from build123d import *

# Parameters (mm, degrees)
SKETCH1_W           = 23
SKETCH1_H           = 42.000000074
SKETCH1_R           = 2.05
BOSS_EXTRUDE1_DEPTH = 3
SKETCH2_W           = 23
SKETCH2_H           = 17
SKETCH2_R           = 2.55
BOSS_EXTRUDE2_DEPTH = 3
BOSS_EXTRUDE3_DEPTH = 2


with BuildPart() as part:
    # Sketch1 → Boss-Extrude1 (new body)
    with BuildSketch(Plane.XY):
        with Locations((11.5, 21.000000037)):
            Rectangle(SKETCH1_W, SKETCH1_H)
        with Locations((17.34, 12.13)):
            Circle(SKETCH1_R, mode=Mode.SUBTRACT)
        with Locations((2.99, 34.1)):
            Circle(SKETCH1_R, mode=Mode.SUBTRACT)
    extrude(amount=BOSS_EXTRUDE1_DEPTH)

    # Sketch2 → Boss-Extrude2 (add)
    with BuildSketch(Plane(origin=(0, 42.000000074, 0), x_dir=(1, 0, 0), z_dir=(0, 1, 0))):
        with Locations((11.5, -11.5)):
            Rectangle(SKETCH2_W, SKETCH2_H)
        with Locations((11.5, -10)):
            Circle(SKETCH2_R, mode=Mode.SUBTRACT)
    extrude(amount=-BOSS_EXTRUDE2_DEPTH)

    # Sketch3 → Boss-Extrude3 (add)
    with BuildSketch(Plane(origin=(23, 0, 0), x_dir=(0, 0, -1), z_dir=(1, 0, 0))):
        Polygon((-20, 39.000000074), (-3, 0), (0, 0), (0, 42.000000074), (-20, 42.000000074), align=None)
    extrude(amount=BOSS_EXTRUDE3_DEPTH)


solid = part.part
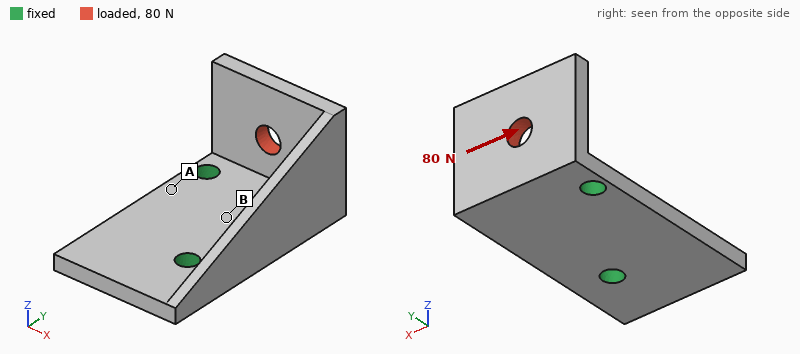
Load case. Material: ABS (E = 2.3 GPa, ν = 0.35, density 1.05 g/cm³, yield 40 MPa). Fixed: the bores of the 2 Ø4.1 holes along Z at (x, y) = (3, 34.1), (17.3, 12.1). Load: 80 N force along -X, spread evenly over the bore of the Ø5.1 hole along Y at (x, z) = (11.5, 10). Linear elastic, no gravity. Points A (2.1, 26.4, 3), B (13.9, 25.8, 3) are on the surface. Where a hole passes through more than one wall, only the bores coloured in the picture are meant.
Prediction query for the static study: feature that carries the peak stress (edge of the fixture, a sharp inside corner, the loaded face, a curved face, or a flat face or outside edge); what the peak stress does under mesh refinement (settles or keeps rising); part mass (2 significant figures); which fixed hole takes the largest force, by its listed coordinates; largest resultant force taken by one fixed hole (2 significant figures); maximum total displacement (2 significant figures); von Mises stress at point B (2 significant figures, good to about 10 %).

edge of the fixture
keeps rising
5.2 g
(3, 34.1)
87 N
0.62 mm
4.1 MPa
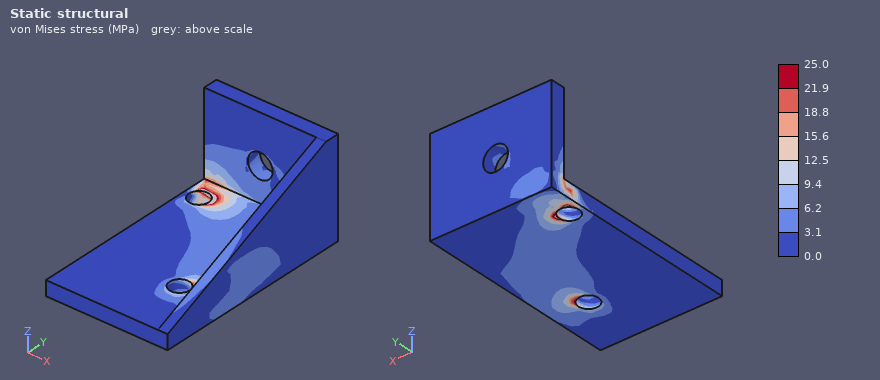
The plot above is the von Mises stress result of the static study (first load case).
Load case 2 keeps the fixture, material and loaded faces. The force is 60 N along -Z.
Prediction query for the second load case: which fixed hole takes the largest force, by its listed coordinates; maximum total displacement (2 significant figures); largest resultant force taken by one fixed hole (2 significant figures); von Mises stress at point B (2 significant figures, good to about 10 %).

(3, 34.1)
0.46 mm
56 N
3.2 MPa
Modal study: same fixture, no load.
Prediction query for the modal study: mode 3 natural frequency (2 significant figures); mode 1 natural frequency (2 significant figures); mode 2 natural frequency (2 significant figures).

2700 Hz
1100 Hz
2200 Hz
